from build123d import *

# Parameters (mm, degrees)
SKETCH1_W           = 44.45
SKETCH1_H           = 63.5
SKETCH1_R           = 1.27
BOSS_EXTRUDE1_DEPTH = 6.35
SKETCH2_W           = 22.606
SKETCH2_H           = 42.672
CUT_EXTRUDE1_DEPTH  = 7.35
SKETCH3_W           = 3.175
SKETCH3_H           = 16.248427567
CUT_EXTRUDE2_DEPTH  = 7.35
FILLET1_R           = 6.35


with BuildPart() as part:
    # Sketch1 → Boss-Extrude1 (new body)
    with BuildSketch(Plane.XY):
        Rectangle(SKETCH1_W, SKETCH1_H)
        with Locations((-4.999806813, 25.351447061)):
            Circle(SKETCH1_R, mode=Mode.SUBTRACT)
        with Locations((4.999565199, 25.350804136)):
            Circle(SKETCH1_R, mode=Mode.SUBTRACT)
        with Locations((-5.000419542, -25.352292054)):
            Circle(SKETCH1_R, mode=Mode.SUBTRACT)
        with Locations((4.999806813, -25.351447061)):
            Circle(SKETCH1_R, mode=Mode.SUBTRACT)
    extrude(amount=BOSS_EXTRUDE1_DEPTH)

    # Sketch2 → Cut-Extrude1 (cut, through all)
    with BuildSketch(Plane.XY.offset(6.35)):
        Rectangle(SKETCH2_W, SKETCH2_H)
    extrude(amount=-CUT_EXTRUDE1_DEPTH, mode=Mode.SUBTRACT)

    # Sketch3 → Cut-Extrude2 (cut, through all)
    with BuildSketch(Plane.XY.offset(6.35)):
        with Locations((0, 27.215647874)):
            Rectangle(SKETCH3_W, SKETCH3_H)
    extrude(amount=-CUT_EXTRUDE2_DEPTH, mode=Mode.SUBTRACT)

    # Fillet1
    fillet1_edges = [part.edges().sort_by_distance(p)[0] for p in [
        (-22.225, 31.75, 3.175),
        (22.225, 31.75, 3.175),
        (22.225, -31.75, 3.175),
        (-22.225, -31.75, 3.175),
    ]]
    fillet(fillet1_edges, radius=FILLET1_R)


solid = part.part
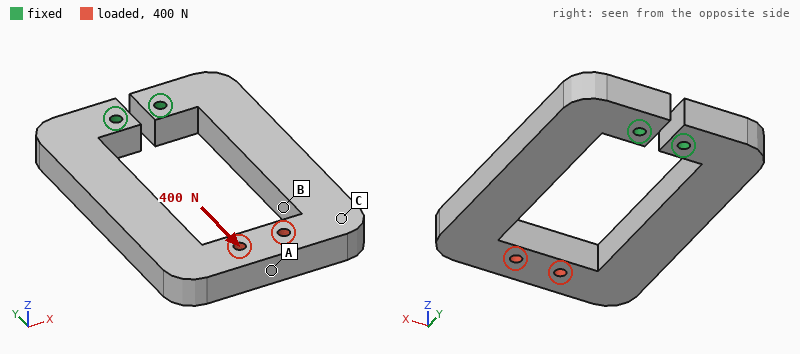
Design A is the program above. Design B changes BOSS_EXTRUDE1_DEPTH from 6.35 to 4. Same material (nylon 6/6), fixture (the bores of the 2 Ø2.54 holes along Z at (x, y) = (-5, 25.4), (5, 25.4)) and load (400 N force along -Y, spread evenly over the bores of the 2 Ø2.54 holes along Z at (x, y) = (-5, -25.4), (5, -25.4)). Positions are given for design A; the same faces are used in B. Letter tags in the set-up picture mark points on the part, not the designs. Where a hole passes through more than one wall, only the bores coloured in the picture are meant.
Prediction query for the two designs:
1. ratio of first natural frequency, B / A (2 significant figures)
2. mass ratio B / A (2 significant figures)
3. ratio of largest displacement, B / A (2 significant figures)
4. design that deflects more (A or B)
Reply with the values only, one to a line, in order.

0.67
0.63
1.6
B
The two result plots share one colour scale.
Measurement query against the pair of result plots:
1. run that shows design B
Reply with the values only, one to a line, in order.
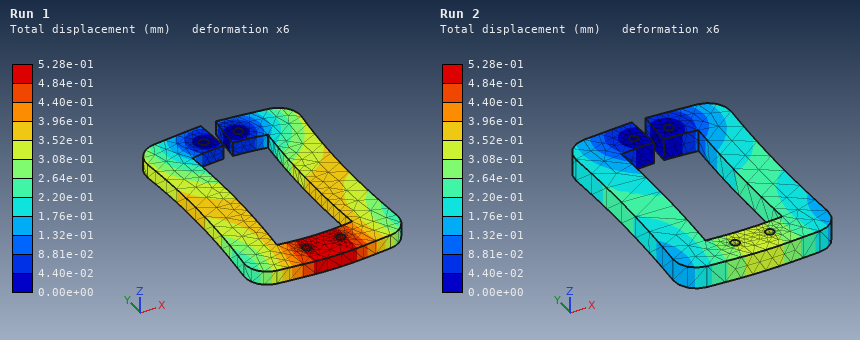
Run 1
